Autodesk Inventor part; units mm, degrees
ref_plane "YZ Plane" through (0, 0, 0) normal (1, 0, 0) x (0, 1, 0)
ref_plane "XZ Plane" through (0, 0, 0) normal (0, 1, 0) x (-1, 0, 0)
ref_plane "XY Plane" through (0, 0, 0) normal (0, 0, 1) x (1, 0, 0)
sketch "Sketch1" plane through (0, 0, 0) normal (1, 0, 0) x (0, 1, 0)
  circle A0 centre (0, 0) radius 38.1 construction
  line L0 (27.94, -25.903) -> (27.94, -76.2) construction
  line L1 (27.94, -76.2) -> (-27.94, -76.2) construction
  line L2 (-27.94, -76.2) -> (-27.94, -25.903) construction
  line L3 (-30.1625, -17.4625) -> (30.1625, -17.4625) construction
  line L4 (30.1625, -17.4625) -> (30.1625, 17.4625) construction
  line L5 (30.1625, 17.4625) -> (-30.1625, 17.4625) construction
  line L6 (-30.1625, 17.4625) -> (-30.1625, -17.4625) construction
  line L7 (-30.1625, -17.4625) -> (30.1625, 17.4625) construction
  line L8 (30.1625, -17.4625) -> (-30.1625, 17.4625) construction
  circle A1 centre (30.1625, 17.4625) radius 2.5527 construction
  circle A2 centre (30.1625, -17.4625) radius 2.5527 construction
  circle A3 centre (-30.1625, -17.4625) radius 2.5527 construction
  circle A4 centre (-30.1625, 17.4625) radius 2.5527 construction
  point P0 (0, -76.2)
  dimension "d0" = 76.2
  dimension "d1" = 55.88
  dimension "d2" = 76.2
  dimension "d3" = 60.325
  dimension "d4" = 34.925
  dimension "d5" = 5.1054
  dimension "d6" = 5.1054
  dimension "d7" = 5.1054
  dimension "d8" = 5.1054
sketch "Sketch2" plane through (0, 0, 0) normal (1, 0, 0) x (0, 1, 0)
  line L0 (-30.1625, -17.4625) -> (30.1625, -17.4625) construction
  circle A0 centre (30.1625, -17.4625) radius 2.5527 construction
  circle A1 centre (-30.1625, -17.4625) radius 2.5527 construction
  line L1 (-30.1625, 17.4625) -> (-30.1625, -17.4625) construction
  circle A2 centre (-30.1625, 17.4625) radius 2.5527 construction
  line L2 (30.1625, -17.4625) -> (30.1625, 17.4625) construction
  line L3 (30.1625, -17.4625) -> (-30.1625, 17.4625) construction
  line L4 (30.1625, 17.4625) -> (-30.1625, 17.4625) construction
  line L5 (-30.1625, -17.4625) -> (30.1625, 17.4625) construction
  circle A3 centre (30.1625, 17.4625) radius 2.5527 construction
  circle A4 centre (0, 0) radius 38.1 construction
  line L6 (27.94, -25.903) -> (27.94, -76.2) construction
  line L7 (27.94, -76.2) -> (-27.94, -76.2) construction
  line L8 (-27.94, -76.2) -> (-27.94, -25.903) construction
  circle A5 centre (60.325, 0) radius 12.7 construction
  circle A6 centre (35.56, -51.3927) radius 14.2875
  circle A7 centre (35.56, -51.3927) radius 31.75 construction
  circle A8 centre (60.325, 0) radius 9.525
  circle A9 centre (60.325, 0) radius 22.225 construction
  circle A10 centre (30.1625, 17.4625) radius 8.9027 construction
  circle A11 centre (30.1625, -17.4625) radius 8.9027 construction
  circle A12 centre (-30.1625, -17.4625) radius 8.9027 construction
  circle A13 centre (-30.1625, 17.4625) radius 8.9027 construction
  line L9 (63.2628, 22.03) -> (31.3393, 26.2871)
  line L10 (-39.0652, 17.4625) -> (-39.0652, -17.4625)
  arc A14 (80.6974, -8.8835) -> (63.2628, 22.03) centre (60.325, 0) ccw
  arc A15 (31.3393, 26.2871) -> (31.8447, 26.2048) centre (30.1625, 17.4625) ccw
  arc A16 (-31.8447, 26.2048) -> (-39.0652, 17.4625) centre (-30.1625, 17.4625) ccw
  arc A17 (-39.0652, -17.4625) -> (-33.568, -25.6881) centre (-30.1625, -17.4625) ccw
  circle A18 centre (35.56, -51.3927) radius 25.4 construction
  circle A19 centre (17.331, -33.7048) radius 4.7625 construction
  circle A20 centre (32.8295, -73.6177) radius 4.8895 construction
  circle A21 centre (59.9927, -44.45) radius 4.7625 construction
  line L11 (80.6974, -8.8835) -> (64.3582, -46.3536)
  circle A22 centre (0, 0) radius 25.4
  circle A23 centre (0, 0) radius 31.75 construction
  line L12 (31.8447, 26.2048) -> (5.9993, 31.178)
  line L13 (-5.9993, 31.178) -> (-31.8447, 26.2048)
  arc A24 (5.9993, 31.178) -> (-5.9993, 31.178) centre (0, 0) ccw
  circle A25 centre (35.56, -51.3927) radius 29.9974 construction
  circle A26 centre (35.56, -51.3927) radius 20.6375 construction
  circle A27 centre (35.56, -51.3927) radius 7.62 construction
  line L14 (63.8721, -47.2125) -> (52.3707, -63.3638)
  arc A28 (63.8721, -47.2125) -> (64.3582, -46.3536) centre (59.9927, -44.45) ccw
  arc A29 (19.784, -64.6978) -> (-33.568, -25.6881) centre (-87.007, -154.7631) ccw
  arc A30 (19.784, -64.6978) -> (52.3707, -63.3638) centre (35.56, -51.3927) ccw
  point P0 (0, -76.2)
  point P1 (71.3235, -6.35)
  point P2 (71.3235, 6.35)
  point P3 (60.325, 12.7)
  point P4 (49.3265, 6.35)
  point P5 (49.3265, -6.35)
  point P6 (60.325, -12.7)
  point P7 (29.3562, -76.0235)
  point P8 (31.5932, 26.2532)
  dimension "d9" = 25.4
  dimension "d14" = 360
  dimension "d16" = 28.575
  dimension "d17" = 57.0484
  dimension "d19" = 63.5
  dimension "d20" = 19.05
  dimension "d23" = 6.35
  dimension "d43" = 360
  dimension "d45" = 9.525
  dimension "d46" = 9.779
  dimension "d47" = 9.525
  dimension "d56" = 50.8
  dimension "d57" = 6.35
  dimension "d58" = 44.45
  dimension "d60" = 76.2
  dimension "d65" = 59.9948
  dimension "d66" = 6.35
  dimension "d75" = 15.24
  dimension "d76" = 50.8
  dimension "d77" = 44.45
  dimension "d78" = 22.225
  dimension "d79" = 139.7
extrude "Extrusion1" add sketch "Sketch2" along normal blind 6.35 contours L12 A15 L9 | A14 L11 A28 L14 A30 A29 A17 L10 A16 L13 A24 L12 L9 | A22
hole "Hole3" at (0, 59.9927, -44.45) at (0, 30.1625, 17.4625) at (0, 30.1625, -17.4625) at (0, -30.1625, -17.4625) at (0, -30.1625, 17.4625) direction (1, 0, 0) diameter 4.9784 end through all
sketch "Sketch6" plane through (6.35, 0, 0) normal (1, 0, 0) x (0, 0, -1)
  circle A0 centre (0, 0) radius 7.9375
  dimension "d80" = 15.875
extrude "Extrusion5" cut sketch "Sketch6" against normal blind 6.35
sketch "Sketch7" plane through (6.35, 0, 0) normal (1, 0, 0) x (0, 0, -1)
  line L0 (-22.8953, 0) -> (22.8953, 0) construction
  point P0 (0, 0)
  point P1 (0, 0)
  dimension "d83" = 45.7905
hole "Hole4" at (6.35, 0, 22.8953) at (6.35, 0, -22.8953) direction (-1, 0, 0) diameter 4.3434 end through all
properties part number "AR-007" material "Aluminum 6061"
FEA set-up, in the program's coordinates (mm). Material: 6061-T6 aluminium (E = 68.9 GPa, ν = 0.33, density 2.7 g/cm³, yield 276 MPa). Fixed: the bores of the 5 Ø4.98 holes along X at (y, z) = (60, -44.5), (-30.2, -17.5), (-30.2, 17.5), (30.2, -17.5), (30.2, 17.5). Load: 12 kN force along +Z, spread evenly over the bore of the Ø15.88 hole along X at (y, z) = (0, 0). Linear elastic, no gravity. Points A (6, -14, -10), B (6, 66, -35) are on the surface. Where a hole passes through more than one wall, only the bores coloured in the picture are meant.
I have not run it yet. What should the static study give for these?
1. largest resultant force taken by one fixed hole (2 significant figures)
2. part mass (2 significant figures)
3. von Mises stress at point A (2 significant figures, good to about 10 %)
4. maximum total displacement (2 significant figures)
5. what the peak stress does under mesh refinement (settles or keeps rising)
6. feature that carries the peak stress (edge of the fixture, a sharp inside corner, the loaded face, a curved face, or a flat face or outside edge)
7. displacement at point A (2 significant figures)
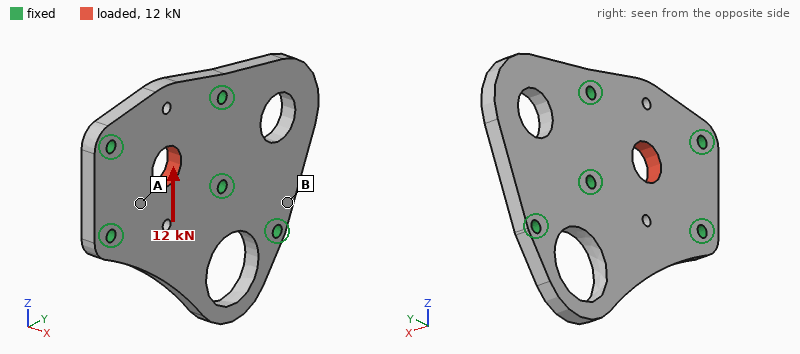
3.5 kN
130 g
31 MPa
24 µm
keeps rising
edge of the fixture
13 µm
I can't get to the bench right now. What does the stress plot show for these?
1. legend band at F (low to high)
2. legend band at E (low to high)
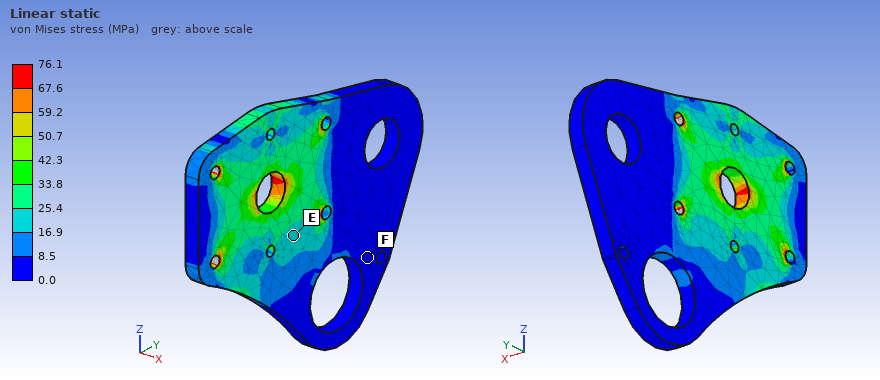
0.0 to 8.5 MPa
16.9 to 25.4 MPa
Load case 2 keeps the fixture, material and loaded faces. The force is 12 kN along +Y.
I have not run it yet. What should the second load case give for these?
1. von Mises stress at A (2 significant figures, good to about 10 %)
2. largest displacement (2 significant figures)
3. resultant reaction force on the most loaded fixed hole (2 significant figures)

28 MPa
13 µm
3.2 kN
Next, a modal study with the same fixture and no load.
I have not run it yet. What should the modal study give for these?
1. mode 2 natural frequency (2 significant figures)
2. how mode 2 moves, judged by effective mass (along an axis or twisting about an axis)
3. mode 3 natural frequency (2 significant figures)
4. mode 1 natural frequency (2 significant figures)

3600 Hz
along X
6600 Hz
3100 Hz
